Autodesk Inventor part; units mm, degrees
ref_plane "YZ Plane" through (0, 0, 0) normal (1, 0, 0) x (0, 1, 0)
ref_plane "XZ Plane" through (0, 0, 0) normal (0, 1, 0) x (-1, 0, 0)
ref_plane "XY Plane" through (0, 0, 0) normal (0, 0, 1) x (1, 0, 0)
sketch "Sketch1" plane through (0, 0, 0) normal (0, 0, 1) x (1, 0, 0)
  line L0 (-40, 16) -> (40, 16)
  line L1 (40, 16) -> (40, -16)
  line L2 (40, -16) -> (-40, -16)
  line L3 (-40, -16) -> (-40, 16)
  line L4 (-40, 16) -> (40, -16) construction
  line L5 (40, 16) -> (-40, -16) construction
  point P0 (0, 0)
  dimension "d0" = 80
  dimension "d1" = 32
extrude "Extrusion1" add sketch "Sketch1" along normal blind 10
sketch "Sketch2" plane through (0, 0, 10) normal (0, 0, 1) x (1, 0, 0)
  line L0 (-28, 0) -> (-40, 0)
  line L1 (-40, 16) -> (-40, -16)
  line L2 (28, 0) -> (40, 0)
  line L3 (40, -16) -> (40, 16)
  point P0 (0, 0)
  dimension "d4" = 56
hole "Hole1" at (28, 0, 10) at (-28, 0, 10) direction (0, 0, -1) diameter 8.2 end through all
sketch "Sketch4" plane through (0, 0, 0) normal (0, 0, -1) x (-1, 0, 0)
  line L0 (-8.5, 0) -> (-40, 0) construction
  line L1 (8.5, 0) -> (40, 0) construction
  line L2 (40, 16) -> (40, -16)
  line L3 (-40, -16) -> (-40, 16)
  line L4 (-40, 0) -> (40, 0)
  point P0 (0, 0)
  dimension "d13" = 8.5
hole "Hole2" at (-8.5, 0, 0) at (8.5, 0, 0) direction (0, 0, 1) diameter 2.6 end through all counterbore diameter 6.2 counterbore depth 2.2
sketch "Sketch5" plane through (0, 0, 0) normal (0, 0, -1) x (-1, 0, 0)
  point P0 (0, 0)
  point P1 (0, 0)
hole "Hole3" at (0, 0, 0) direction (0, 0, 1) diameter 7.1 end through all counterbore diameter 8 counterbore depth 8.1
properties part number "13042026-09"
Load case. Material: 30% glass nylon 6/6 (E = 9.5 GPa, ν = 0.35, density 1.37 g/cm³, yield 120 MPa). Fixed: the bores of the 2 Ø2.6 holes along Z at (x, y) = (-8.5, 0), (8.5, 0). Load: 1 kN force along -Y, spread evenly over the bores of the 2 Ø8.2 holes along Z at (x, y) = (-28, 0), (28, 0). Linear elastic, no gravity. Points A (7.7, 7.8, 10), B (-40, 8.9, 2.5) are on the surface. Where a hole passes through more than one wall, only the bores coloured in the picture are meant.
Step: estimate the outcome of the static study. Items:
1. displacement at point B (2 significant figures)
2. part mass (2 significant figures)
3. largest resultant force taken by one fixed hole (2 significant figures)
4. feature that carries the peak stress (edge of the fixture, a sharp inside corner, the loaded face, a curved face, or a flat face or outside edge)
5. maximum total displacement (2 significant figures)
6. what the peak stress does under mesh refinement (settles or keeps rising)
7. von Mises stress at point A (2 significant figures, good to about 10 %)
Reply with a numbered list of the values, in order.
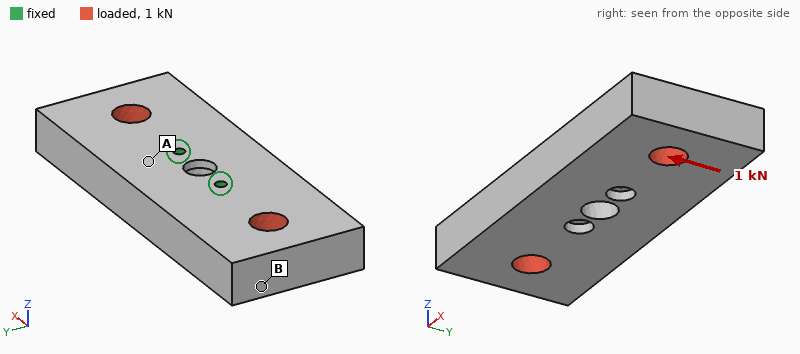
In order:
1. 37 µm
2. 33 g
3. 500 N
4. edge of the fixture
5. 40 µm
6. keeps rising
7. 3.2 MPa
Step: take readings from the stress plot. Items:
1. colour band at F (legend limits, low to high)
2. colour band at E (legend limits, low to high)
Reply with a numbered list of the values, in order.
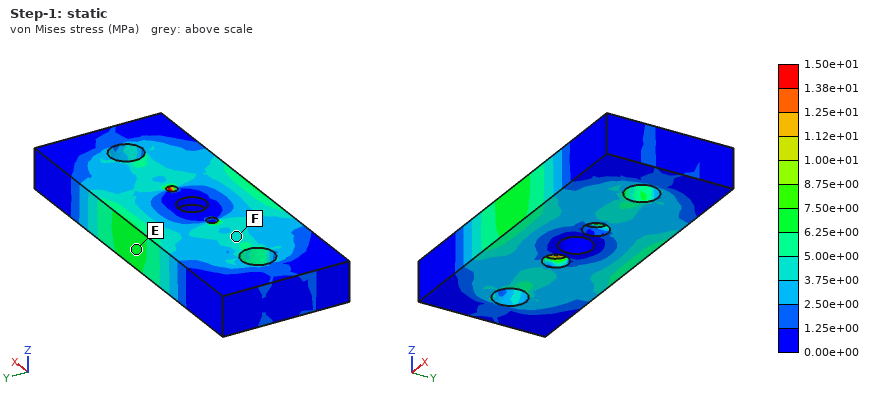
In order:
1. 3.75e+00 to 5.00e+00 MPa
2. 6.25e+00 to 7.50e+00 MPa
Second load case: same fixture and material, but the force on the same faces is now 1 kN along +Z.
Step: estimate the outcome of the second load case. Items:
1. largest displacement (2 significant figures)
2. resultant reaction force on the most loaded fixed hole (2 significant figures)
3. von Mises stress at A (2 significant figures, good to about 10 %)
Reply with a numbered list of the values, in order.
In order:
1. 0.18 mm
2. 550 N
3. 13 MPa
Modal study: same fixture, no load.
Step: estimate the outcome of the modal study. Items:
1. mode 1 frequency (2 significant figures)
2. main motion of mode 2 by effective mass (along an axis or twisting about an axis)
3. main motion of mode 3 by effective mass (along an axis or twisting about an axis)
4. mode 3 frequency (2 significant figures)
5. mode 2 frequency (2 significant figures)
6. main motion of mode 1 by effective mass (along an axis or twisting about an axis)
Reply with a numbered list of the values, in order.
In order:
1. 2900 Hz
2. along Z
3. twisting about Z
4. 3900 Hz
5. 3100 Hz
6. twisting about Y
